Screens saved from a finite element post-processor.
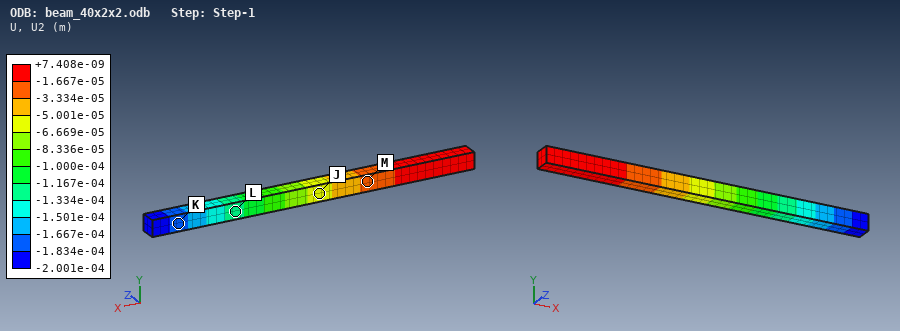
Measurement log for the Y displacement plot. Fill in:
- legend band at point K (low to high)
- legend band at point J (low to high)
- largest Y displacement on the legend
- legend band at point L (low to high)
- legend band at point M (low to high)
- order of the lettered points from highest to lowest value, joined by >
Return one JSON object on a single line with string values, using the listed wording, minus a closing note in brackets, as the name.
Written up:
{"legend band at point K": "-1.834e-04 to -1.667e-04 m", "legend band at point J": "-6.669e-05 to -5.001e-05 m", "largest Y displacement on the legend": "+7.408e-09 m", "legend band at point L": "-1.334e-04 to -1.167e-04 m", "legend band at point M": "-3.334e-05 to -1.667e-05 m", "order of the lettered points from highest to lowest value, joined by >": "M > J > L > K"}
